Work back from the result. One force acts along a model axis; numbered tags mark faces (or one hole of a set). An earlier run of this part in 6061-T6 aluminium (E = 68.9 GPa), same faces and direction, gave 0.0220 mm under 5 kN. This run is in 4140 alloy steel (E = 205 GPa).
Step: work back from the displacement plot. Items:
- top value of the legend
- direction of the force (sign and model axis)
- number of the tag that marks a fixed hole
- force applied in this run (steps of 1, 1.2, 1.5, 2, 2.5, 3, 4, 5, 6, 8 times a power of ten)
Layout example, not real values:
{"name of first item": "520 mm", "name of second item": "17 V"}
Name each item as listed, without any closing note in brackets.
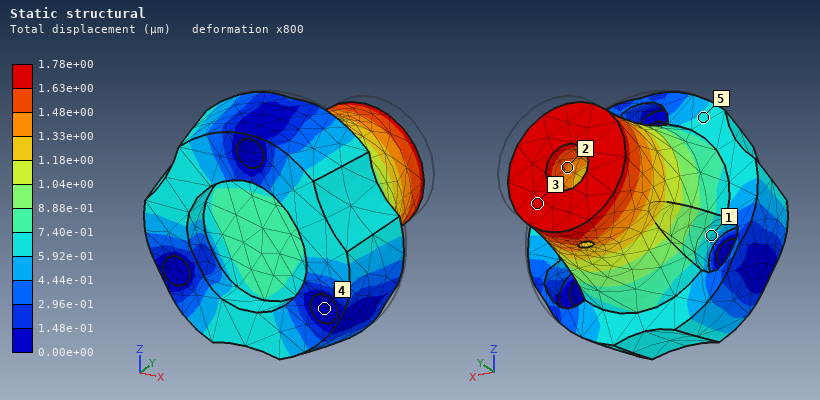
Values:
{"top value of the legend": "1.78e+00 µm", "direction of the force": "-Y", "number of the tag that marks a fixed hole": "4", "force applied in this run": "1.2 kN"}
